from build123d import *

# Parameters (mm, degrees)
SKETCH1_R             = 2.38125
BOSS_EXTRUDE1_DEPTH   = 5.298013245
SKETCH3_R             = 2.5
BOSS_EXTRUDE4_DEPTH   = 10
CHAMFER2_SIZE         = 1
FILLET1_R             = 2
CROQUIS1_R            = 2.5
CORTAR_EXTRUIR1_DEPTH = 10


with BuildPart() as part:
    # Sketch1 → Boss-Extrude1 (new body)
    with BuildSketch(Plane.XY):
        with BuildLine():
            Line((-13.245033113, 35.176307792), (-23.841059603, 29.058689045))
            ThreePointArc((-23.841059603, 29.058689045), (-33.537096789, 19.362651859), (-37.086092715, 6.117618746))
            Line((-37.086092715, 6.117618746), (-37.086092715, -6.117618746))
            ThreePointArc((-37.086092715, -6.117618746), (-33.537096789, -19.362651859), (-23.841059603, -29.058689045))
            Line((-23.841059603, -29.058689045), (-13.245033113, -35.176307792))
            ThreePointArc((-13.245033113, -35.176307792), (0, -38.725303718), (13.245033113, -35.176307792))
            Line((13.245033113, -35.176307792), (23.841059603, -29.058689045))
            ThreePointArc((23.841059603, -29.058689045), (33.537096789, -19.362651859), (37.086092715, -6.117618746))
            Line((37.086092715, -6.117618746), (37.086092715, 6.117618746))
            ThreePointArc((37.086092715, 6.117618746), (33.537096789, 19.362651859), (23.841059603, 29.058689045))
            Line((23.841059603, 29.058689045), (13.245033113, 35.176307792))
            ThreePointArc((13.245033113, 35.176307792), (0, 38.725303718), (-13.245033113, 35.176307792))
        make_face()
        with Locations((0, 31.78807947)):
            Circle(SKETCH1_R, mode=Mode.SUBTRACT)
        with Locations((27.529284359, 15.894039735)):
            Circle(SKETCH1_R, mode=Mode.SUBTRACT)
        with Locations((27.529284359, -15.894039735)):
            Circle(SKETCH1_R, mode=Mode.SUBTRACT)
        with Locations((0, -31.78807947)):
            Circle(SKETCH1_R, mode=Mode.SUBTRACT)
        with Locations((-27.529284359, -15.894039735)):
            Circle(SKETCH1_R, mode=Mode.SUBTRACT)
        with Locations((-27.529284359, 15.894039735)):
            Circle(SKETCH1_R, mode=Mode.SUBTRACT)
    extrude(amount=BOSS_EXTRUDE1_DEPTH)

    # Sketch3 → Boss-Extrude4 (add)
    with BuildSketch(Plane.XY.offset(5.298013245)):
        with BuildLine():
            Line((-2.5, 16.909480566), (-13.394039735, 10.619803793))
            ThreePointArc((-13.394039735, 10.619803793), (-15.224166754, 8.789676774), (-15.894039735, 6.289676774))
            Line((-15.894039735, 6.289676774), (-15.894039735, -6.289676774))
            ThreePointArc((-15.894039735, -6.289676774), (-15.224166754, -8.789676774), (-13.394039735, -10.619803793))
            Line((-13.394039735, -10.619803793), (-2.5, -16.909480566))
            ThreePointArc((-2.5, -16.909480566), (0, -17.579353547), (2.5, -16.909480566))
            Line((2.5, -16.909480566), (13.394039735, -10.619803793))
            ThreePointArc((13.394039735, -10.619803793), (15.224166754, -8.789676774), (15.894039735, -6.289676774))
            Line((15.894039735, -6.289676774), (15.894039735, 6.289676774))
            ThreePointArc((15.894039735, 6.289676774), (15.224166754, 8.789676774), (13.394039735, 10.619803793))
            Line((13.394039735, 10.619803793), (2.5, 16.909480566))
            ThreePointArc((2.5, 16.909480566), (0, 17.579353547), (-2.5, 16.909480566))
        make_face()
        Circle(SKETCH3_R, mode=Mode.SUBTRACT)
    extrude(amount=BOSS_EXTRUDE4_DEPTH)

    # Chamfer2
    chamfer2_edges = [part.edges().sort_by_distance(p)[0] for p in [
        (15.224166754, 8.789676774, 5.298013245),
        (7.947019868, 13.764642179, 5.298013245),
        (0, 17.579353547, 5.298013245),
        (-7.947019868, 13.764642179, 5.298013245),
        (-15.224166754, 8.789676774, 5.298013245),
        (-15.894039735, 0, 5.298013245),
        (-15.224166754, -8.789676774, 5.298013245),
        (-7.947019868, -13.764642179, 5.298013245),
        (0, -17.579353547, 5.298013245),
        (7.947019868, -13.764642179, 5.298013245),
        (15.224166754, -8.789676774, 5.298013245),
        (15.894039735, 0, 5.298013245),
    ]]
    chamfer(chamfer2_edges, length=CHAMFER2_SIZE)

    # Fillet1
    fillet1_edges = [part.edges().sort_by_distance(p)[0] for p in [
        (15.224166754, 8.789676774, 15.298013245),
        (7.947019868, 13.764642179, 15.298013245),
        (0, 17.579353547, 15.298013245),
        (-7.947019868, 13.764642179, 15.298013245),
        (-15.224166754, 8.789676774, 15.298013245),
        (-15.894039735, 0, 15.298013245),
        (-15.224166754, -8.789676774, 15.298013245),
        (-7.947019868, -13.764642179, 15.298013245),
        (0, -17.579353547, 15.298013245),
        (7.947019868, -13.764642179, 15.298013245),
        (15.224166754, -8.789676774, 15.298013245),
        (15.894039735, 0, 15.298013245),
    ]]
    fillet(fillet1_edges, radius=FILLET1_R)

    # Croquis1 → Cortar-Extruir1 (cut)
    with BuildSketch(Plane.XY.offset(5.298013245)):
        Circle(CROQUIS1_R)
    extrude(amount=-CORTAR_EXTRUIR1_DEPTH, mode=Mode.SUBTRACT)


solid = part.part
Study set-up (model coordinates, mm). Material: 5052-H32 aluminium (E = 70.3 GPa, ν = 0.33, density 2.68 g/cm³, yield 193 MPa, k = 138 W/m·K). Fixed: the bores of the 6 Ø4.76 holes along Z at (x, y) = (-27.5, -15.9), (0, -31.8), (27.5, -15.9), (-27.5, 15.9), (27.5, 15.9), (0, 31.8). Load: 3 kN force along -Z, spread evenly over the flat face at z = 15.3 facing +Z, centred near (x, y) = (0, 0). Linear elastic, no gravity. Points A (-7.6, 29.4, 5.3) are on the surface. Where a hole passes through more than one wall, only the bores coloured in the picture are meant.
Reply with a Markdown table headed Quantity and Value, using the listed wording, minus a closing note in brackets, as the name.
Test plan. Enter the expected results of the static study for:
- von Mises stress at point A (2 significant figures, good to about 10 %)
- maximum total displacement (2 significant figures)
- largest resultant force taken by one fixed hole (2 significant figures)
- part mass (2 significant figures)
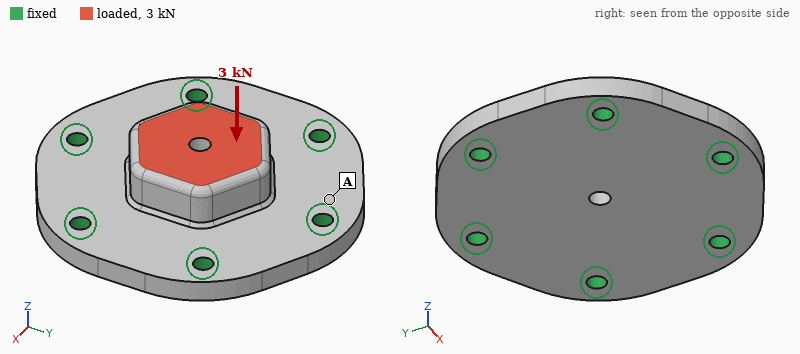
| Quantity | Value |
|---|---|
| von Mises stress at point A | 11 MPa |
| maximum total displacement | 17 µm |
| largest resultant force taken by one fixed hole | 550 N |
| part mass | 85 g |
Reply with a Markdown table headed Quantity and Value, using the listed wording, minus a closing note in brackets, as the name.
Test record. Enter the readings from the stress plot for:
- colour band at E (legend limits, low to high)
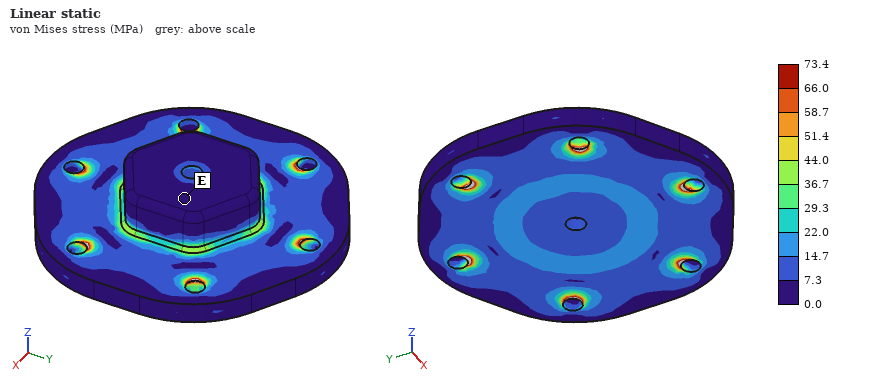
| Quantity | Value |
|---|---|
| colour band at E | 0.0 to 7.3 MPa |
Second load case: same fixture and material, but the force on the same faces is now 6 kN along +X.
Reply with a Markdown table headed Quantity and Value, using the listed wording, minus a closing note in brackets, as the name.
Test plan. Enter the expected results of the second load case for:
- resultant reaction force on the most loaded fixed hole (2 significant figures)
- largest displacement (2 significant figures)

| Quantity | Value |
|---|---|
| resultant reaction force on the most loaded fixed hole | 1.6 kN |
| largest displacement | 27 µm |
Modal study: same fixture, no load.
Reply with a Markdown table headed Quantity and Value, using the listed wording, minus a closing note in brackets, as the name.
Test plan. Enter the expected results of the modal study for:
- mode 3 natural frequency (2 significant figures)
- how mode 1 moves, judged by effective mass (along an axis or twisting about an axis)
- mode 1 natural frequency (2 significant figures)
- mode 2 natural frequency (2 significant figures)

| Quantity | Value |
|---|---|
| mode 3 natural frequency | 17 kHz |
| how mode 1 moves, judged by effective mass | along Z |
| mode 1 natural frequency | 11 kHz |
| mode 2 natural frequency | 17 kHz |
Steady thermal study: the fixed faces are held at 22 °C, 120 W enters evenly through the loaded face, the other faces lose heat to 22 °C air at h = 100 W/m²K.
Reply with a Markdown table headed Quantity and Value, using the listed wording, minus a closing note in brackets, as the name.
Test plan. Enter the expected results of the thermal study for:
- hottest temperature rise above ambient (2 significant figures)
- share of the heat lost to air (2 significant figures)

| Quantity | Value |
|---|---|
| hottest temperature rise above ambient | 37 K |
| share of the heat lost to air | 9.6 % |
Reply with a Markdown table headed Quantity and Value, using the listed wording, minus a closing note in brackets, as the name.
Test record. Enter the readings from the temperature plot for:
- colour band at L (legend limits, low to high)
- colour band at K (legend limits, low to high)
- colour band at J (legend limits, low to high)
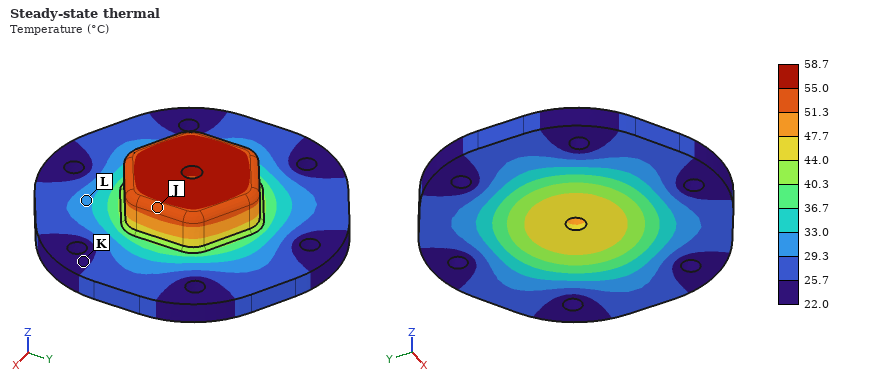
| Quantity | Value |
|---|---|
| colour band at L | 29.3 to 33.0 °C |
| colour band at K | 22.0 to 25.7 °C |
| colour band at J | 51.3 to 55.0 °C |
